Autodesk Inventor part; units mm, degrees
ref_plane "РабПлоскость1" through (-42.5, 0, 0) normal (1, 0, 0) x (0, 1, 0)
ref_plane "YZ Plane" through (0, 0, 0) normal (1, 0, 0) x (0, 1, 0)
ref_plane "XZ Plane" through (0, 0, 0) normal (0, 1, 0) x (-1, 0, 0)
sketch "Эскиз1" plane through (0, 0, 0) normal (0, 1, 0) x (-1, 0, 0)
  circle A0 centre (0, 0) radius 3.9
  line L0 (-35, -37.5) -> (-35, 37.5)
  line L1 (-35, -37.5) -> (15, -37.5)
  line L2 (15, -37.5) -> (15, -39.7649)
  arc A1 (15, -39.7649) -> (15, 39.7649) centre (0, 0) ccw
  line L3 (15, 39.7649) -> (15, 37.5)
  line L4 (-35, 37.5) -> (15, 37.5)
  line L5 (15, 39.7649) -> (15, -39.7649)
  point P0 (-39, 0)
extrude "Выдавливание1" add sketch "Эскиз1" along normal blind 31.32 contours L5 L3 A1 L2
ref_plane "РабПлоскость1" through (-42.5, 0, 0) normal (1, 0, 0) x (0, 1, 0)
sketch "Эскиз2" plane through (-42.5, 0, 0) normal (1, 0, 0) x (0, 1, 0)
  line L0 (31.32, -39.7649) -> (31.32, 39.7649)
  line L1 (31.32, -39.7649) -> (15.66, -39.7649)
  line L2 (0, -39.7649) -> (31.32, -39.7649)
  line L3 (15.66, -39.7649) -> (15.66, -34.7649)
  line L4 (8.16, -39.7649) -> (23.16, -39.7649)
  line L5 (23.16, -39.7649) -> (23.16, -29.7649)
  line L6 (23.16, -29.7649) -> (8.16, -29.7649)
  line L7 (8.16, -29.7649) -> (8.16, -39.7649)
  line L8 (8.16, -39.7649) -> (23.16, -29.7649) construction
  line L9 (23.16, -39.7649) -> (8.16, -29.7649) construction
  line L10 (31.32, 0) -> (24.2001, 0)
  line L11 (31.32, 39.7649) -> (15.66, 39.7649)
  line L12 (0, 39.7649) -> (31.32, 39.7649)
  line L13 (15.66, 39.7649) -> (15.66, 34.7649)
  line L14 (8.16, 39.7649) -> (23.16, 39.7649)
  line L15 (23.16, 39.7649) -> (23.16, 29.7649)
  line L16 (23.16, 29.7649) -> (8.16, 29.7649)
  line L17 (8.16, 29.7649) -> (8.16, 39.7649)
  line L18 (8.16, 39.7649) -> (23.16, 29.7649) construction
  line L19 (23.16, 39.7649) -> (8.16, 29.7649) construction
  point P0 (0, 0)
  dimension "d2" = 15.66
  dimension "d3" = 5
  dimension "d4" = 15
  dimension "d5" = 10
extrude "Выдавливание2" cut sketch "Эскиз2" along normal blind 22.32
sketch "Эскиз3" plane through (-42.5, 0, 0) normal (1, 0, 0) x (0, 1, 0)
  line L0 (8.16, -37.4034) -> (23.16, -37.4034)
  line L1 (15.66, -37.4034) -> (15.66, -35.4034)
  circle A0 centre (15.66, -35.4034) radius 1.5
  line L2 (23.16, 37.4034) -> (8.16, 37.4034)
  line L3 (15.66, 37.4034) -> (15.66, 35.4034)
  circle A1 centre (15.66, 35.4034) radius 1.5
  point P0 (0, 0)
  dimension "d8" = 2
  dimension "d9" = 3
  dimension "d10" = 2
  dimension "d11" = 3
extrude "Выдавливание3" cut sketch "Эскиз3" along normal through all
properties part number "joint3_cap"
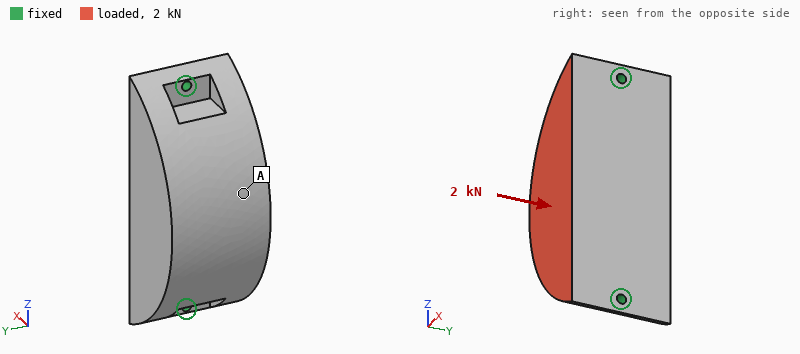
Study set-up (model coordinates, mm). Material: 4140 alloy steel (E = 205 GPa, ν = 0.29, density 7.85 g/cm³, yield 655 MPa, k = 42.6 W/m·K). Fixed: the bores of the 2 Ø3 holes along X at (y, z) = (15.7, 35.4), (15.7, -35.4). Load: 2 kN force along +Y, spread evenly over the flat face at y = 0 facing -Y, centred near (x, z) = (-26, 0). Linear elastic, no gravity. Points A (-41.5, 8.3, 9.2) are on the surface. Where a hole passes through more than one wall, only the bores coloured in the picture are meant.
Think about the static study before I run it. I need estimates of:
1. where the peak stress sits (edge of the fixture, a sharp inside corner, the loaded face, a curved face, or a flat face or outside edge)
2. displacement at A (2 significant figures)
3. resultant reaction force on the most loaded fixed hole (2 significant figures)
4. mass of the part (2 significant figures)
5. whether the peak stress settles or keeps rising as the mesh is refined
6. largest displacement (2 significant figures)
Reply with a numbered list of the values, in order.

1. edge of the fixture
2. 25 µm
3. 1.0 kN
4. 380 g
5. keeps rising
6. 30 µm
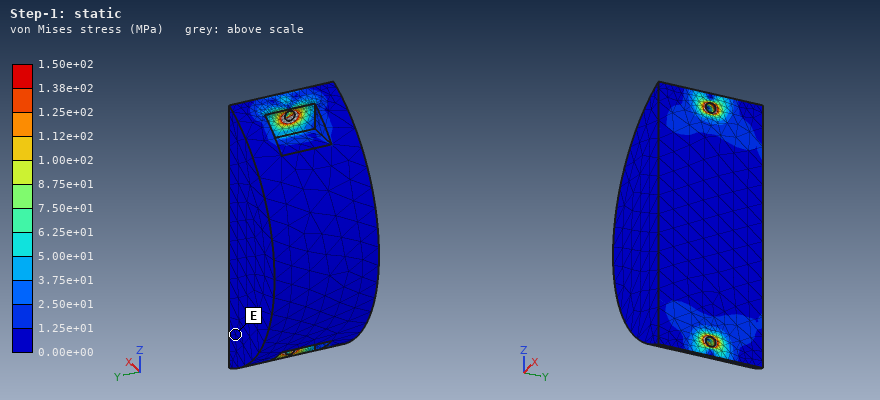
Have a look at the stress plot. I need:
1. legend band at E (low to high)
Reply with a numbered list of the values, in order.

1. 0.00e+00 to 1.25e+01 MPa
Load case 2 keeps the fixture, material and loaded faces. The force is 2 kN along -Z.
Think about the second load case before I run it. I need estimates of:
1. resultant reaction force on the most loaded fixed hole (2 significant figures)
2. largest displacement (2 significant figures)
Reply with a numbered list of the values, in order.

1. 1.1 kN
2. 1.7 µm
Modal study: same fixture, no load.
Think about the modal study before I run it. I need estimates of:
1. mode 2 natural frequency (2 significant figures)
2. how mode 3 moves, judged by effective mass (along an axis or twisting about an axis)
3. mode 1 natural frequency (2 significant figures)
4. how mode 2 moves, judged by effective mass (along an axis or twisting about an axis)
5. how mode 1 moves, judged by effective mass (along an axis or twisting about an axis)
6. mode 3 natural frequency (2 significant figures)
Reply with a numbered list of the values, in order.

1. 6800 Hz
2. along Z
3. 2400 Hz
4. along X
5. along Y
6. 11 kHz
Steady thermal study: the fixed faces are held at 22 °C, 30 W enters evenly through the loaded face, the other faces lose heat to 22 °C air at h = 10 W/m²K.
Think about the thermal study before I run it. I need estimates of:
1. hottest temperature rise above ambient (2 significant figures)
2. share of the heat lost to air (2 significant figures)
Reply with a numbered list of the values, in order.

1. 41 K
2. 7.6 %
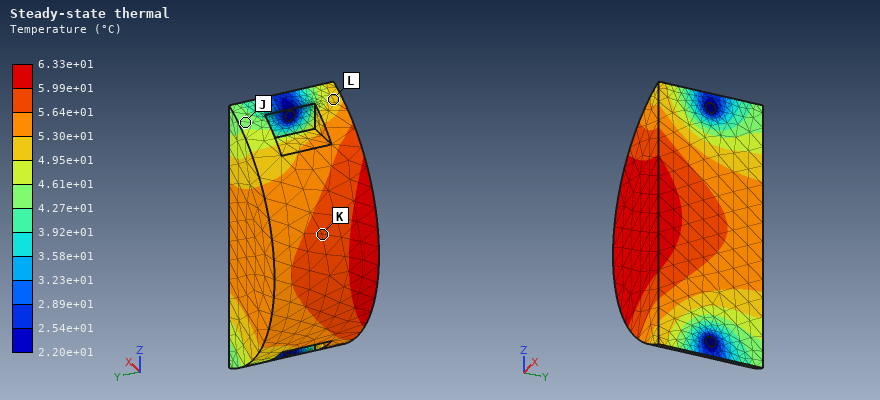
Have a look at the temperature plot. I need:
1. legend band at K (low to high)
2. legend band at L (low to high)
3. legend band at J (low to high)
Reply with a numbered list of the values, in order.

1. 5.64e+01 to 5.99e+01 °C
2. 4.95e+01 to 5.30e+01 °C
3. 4.27e+01 to 4.61e+01 °C
